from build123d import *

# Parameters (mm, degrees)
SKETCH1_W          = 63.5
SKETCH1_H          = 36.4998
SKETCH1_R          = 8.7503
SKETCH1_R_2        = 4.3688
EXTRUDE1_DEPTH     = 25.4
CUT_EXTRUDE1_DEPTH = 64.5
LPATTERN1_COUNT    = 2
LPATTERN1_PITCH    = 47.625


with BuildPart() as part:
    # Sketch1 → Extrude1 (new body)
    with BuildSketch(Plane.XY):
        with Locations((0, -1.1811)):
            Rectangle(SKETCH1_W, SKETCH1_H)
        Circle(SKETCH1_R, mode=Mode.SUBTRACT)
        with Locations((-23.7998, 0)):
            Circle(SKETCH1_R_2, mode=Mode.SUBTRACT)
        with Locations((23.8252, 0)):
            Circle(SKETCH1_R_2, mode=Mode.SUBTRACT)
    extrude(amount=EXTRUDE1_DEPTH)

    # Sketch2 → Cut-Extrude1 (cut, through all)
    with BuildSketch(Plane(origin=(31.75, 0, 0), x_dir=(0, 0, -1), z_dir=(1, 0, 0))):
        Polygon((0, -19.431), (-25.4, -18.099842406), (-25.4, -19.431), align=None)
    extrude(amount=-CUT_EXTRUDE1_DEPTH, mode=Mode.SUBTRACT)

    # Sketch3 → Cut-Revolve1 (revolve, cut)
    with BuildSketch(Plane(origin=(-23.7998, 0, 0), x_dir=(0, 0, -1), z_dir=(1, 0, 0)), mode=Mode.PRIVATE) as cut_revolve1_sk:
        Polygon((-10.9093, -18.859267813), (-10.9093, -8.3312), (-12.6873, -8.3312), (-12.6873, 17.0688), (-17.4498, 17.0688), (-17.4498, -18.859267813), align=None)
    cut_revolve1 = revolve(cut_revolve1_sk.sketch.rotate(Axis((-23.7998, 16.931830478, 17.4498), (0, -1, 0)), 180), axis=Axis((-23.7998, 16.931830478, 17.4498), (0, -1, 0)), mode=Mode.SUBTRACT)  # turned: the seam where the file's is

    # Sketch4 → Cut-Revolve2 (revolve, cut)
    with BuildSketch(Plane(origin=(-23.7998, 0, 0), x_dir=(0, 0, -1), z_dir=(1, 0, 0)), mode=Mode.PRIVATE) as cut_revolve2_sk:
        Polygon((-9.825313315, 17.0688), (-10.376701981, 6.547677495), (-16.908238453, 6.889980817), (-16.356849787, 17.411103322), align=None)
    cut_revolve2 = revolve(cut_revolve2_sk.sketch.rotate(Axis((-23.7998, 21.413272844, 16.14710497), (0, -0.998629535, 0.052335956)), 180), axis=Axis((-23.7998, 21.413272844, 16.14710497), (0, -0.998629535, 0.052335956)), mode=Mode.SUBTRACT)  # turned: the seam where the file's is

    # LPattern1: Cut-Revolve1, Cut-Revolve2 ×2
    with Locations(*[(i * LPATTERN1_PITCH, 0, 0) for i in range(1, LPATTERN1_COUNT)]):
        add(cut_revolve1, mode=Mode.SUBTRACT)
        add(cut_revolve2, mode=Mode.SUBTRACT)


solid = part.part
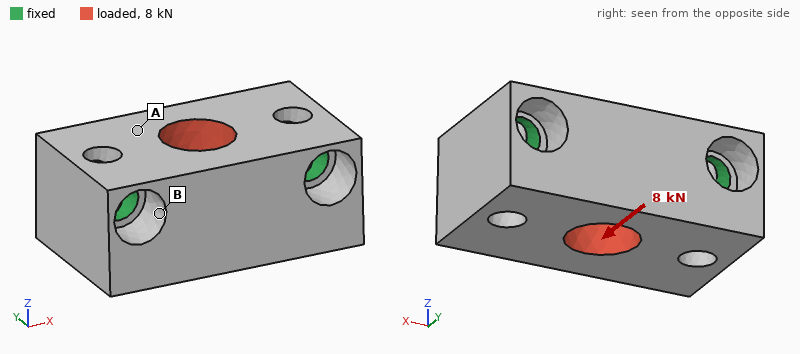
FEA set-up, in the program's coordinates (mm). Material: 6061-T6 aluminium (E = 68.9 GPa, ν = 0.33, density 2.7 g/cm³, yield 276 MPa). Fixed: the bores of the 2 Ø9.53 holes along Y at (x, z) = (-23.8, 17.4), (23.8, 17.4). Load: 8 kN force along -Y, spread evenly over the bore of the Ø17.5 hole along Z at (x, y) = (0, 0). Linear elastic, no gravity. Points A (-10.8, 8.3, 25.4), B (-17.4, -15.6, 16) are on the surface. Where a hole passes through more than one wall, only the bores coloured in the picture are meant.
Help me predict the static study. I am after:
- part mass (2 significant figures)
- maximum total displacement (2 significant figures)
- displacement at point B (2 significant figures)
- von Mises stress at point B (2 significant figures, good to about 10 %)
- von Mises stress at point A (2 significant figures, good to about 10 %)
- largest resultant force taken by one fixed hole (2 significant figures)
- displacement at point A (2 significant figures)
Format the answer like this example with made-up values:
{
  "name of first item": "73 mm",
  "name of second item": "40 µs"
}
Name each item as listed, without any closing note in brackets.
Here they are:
{
  "part mass": "110 g",
  "maximum total displacement": "12 µm",
  "displacement at point B": "4.8 µm",
  "von Mises stress at point B": "5.1 MPa",
  "von Mises stress at point A": "9.3 MPa",
  "largest resultant force taken by one fixed hole": "4.0 kN",
  "displacement at point A": "3.2 µm"
}
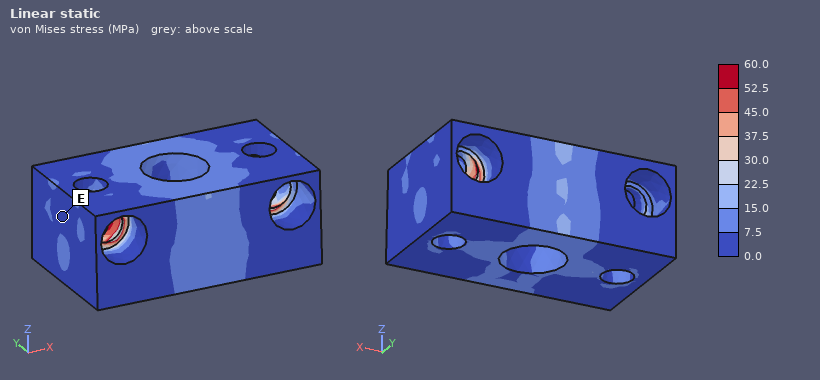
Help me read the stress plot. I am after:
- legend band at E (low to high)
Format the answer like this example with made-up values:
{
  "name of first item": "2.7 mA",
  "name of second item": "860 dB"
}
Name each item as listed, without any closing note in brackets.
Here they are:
{
  "legend band at E": "0.0 to 7.5 MPa"
}
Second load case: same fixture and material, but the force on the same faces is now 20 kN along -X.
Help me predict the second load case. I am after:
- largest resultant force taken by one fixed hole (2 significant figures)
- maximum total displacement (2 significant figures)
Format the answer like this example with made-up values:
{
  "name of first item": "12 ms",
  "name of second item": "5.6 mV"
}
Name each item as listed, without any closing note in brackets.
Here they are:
{
  "largest resultant force taken by one fixed hole": "10 kN",
  "maximum total displacement": "10.0 µm"
}
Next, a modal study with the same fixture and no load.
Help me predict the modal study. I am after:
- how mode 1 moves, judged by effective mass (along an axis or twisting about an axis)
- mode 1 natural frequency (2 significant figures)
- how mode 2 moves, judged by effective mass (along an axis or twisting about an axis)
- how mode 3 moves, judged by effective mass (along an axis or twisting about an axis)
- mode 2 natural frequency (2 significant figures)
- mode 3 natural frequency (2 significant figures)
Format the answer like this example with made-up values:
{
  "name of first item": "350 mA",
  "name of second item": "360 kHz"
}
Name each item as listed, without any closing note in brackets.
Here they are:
{
  "how mode 1 moves, judged by effective mass": "along Y",
  "mode 1 natural frequency": "13 kHz",
  "how mode 2 moves, judged by effective mass": "along Z",
  "how mode 3 moves, judged by effective mass": "twisting about Z",
  "mode 2 natural frequency": "19 kHz",
  "mode 3 natural frequency": "23 kHz"
}
